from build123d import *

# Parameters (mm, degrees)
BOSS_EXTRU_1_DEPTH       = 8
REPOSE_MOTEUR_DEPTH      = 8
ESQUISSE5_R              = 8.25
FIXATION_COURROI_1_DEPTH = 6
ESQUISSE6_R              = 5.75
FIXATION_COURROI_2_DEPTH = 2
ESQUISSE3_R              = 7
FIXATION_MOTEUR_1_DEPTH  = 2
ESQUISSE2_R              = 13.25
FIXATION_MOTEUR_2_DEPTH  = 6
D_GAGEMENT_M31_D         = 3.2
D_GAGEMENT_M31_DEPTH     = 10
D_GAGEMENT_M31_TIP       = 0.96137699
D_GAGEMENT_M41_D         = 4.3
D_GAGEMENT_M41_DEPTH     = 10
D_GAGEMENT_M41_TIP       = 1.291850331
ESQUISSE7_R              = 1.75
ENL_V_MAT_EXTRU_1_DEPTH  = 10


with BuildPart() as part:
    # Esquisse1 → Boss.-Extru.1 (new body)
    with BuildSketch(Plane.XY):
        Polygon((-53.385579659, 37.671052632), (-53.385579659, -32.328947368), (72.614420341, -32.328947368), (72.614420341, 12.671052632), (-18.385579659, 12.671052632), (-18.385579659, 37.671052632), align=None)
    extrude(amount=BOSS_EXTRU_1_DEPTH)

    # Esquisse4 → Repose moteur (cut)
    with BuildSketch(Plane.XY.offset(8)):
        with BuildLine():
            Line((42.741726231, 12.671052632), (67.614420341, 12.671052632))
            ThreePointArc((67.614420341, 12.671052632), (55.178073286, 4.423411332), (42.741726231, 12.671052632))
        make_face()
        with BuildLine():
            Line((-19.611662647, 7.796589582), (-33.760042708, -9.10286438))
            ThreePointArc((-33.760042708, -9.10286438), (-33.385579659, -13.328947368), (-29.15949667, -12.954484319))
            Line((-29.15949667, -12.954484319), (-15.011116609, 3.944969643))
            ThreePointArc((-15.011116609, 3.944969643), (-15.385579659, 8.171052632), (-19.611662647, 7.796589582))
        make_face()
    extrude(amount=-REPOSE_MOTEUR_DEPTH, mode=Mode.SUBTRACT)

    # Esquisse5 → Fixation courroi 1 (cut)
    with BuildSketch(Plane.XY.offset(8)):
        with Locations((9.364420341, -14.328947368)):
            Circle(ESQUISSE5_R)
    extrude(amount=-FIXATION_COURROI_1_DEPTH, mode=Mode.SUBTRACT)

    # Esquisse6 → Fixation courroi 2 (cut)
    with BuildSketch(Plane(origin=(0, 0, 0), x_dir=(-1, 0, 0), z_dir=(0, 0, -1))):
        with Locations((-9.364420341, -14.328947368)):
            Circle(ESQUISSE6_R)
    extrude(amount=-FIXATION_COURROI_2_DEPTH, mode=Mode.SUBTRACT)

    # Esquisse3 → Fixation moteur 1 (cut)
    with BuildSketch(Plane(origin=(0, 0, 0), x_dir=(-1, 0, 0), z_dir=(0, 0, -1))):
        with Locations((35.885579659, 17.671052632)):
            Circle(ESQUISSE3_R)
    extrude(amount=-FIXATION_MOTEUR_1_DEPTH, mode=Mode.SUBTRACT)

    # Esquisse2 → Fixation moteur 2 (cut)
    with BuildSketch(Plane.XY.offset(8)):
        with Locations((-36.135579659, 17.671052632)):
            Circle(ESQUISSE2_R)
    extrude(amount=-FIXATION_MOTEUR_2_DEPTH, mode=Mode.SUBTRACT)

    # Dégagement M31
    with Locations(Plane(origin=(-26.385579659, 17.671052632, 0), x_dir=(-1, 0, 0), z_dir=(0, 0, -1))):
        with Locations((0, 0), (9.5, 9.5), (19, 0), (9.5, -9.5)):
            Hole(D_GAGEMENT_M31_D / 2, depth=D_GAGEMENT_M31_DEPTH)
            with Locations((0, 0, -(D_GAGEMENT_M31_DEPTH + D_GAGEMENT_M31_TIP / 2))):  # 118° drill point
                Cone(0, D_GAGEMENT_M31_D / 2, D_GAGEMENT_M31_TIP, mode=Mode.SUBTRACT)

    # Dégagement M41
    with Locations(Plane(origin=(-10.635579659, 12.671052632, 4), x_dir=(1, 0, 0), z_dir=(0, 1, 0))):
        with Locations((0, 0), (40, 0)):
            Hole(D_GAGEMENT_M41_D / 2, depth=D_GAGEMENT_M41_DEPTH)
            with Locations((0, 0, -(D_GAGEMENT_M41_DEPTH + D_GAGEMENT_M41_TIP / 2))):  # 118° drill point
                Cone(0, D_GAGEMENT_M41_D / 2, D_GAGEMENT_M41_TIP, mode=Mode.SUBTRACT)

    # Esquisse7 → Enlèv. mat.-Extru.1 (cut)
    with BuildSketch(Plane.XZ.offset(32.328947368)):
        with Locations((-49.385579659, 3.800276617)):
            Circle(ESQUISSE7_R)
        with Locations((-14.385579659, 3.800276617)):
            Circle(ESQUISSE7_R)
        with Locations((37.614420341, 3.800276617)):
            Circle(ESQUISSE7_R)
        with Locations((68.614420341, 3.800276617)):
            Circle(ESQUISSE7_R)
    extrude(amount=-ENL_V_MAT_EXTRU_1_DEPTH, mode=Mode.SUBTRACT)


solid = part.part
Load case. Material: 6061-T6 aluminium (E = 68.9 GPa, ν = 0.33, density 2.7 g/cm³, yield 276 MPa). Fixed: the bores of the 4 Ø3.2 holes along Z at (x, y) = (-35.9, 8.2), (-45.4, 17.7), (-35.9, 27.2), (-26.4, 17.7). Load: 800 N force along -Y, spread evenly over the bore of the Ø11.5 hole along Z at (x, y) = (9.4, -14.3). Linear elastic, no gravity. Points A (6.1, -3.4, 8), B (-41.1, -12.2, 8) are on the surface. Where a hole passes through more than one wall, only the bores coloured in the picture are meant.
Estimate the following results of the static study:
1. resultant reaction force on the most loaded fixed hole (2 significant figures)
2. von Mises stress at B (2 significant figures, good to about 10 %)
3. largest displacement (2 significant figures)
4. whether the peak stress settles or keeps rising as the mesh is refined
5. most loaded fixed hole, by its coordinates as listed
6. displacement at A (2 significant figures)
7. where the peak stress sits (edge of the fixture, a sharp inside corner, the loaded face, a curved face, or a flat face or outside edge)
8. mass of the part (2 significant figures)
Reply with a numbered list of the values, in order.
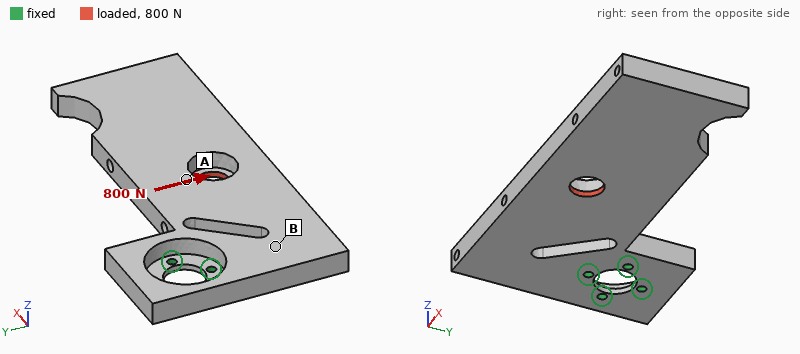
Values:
1. 1.3 kN
2. 15 MPa
3. 0.15 mm
4. keeps rising
5. (-26.4, 17.7)
6. 0.052 mm
7. edge of the fixture
8. 120 g
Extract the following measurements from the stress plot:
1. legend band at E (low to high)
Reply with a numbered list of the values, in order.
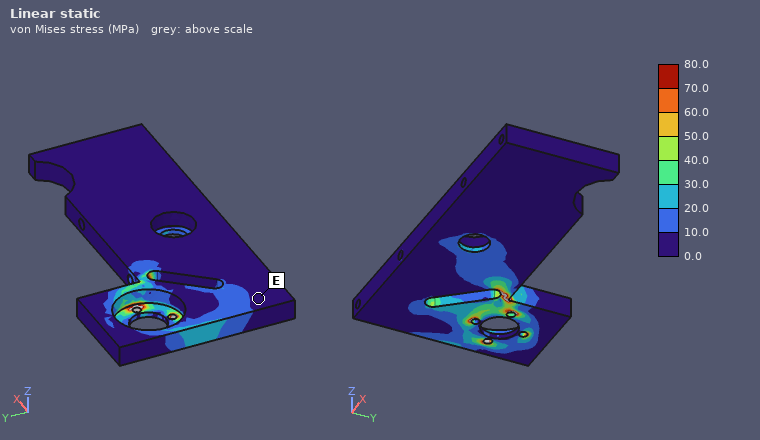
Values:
1. 0.0 to 10.0 MPa
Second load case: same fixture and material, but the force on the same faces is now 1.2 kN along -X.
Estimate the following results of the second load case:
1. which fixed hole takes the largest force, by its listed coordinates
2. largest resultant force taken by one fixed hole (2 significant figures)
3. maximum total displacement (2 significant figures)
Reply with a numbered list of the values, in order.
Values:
1. (-35.9, 8.2)
2. 1.3 kN
3. 0.26 mm
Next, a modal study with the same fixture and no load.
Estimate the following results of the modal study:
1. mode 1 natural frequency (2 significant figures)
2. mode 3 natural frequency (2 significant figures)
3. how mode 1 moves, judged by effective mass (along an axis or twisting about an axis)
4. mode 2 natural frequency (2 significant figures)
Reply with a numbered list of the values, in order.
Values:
1. 330 Hz
2. 1300 Hz
3. along Z
4. 1300 Hz
